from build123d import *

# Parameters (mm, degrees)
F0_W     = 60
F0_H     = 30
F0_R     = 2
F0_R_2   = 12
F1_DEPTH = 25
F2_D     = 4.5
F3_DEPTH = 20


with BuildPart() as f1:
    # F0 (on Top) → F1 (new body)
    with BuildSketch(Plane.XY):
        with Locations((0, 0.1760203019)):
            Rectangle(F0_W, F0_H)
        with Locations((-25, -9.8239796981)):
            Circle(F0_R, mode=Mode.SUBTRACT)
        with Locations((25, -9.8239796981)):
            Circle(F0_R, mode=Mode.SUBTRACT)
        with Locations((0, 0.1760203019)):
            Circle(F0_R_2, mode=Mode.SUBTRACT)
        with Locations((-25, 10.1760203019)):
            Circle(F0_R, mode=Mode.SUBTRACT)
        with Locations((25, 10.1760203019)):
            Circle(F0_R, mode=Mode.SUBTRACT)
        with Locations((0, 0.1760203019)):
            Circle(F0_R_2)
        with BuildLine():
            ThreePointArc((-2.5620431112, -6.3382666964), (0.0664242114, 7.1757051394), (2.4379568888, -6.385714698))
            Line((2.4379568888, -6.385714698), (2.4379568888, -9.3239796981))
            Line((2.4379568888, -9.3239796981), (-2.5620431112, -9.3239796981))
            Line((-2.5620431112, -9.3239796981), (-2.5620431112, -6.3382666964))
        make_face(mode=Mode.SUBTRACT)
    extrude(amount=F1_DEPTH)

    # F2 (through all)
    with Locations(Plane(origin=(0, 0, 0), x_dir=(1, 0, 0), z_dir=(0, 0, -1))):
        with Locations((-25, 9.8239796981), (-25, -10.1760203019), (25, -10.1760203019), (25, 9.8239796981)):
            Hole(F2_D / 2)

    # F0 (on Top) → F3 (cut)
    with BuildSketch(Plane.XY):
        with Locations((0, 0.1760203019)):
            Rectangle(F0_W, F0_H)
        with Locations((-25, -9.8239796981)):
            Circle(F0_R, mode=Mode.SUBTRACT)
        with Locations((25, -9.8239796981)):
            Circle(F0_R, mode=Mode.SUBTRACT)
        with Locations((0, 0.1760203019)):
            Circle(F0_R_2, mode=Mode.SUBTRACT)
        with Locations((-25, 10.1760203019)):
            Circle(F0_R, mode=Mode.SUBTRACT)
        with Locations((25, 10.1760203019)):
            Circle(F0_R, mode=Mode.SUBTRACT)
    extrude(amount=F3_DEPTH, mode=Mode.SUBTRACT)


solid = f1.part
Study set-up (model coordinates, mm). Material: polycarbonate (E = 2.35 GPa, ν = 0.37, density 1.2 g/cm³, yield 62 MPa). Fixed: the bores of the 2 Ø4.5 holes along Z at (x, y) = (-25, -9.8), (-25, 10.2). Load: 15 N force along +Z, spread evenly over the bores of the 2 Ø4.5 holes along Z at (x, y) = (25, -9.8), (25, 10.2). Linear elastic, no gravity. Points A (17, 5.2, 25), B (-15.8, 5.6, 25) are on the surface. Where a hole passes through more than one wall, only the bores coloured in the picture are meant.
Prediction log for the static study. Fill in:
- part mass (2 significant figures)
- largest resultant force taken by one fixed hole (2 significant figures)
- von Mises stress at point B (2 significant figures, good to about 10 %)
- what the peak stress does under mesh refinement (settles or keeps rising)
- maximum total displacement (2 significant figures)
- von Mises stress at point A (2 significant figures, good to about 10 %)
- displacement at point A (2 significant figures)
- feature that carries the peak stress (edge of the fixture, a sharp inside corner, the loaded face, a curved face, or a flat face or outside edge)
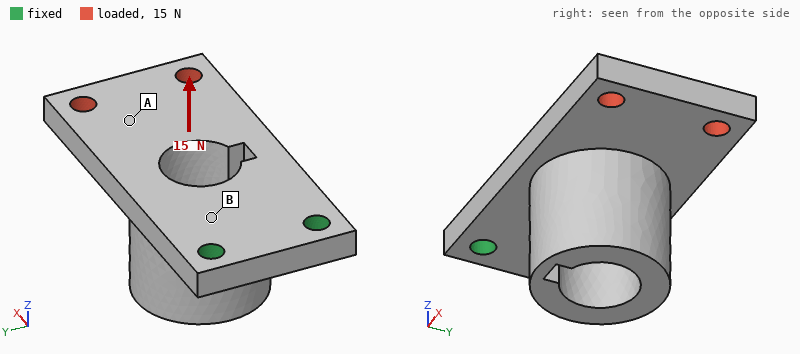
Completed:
16 g
8.6 N
4.3 MPa
keeps rising
0.73 mm
0.85 MPa
0.50 mm
edge of the fixture
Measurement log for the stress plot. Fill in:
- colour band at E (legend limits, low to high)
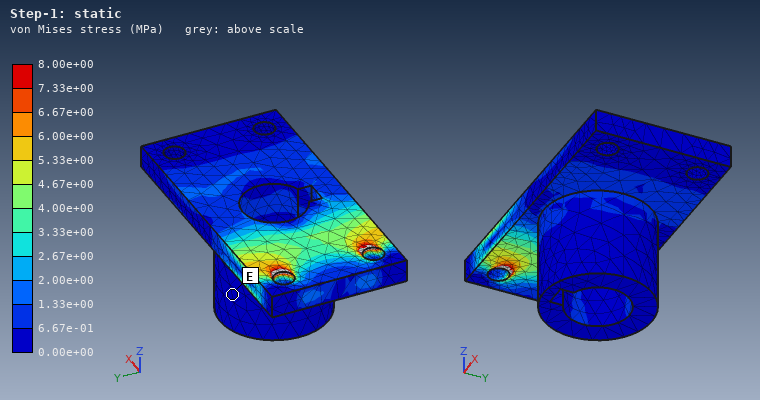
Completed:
0.00e+00 to 6.67e-01 MPa
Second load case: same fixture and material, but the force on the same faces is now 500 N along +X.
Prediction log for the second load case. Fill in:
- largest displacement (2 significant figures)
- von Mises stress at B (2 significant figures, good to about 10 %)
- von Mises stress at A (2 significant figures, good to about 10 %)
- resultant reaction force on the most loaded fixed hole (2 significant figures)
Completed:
0.22 mm
2.7 MPa
2.5 MPa
250 N
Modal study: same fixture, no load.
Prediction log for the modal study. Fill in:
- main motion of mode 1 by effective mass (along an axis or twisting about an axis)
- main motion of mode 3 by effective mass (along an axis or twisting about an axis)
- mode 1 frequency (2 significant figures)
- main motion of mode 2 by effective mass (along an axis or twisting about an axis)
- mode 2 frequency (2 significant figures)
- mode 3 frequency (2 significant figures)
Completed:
along Z
along Y
350 Hz
along Y
1100 Hz
1600 Hz
